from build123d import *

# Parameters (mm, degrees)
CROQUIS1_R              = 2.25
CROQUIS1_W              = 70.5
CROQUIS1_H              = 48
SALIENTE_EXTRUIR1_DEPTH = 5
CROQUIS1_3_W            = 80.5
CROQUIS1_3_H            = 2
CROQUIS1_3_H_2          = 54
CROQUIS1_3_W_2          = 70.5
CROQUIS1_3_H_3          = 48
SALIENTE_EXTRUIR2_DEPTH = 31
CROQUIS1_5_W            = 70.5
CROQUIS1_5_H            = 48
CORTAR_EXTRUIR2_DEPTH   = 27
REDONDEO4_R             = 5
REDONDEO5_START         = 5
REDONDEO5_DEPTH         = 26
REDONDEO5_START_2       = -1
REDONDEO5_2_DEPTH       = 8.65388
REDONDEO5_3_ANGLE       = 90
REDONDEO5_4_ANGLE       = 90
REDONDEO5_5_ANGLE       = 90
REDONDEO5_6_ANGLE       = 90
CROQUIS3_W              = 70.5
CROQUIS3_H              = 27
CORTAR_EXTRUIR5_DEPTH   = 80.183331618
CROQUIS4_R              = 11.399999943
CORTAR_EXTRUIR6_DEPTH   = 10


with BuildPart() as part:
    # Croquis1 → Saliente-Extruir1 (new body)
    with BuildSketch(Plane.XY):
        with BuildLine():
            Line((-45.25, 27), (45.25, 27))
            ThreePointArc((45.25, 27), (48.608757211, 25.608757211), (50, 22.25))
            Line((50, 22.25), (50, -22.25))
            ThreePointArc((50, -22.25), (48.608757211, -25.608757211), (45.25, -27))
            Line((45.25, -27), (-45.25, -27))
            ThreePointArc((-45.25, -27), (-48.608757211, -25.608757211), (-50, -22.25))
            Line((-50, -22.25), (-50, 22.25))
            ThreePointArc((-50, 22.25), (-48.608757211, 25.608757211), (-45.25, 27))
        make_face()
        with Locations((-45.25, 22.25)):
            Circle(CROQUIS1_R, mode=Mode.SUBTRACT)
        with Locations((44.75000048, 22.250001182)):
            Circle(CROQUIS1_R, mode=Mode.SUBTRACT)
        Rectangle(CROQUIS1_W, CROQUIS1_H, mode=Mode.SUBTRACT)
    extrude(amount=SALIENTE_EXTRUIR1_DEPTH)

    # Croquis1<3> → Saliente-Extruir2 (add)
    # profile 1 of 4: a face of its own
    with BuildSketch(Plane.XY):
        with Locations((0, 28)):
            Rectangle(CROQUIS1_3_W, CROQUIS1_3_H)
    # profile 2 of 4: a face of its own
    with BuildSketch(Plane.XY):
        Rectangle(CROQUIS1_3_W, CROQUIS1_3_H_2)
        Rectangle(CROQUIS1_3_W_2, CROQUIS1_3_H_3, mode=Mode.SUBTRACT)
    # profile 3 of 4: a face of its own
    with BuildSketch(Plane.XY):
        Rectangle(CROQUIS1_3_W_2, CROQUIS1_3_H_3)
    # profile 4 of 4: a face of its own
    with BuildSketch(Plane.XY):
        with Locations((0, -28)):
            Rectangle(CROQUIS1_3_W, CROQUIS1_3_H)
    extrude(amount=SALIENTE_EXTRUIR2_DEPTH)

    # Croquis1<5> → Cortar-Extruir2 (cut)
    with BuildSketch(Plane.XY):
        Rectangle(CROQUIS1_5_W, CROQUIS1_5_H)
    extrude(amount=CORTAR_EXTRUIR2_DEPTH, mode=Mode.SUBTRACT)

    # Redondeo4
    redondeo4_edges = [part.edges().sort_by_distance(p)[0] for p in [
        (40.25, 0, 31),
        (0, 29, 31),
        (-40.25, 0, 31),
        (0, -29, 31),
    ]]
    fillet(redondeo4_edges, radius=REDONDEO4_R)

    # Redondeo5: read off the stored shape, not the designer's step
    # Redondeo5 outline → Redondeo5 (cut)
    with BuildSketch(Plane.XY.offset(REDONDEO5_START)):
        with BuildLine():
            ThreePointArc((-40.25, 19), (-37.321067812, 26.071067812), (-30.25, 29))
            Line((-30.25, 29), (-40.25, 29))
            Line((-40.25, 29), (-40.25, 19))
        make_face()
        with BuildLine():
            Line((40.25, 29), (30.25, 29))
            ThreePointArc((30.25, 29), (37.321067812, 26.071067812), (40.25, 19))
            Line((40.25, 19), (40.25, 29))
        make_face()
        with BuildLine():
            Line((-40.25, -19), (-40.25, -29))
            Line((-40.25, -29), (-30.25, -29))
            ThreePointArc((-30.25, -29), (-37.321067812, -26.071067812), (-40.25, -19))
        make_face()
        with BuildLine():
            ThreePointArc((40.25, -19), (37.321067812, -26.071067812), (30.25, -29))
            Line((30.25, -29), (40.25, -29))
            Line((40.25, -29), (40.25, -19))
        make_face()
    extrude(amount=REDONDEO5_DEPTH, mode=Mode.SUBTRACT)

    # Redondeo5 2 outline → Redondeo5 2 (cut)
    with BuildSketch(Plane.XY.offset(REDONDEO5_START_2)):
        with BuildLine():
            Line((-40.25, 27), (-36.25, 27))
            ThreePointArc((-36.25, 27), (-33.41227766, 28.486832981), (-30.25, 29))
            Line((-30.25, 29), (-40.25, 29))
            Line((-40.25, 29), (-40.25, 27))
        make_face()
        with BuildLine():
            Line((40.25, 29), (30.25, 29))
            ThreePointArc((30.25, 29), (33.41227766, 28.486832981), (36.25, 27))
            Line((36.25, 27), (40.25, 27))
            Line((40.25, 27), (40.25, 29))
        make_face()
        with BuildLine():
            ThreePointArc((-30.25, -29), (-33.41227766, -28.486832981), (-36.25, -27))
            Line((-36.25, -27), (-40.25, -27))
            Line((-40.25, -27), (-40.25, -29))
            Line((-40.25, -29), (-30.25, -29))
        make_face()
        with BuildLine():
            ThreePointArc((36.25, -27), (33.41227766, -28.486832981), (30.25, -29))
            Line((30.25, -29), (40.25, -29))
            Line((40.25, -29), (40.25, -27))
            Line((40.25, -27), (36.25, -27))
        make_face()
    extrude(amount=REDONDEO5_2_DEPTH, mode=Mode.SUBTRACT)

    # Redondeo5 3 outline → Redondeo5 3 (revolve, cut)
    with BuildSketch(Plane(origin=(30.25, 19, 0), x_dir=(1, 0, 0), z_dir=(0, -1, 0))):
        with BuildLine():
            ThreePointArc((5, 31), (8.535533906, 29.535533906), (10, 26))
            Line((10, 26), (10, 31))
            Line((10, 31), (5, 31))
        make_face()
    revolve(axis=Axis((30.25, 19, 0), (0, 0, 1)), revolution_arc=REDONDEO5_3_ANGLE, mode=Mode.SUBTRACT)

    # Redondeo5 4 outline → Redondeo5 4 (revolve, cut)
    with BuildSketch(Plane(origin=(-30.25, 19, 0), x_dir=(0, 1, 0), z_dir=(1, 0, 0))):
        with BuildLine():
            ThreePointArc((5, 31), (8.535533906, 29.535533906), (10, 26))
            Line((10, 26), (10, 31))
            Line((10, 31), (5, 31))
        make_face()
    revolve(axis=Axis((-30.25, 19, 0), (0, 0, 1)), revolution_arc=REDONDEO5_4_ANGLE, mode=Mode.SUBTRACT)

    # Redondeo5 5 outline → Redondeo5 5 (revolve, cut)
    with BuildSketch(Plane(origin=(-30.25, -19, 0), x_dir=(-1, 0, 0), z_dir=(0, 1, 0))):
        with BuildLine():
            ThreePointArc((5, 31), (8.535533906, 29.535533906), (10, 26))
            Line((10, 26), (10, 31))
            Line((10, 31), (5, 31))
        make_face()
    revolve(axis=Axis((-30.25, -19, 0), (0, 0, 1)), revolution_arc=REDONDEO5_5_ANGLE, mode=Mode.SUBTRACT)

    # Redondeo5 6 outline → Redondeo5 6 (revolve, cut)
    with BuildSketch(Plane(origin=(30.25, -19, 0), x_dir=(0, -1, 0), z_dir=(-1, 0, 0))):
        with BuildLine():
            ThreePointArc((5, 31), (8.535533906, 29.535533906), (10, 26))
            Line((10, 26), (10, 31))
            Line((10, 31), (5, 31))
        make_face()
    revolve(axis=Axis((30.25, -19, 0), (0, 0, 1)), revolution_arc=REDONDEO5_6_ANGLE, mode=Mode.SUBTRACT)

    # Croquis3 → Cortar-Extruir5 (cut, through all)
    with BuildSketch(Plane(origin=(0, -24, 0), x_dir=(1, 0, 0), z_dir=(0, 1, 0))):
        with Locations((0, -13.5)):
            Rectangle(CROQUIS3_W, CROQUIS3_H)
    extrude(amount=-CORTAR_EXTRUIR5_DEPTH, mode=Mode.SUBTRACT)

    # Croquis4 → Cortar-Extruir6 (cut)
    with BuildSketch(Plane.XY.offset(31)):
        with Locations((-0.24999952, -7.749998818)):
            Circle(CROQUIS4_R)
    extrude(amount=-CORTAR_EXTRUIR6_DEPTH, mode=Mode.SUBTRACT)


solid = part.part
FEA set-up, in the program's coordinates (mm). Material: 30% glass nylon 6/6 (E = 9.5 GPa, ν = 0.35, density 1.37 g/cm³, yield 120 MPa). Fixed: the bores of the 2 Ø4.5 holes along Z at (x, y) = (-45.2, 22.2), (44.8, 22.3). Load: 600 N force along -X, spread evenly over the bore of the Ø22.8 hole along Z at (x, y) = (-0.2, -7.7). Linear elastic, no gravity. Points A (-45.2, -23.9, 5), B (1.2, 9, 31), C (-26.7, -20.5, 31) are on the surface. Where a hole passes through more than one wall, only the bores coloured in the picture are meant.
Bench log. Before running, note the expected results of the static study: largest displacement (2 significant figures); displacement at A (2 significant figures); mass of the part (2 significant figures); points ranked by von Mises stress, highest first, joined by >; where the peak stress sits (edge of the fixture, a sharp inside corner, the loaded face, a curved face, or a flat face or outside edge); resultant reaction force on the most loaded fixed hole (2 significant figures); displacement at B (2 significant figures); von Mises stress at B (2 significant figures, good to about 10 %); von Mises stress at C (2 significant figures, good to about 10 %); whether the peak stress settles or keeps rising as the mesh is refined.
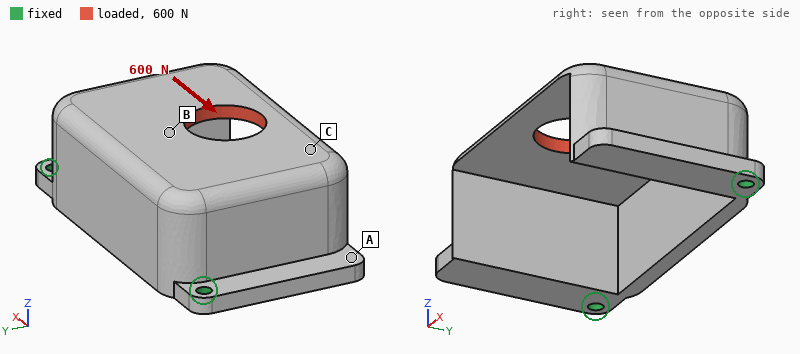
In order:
0.63 mm
0.38 mm
60 g
C > B > A
edge of the fixture
390 N
0.14 mm
7.2 MPa
12 MPa
keeps rising
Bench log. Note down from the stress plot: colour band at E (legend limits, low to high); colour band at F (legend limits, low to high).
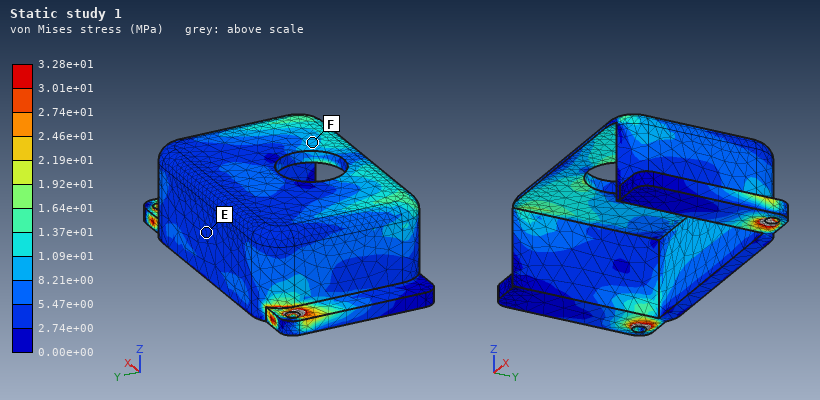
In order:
2.74e+00 to 5.47e+00 MPa
8.21e+00 to 1.09e+01 MPa
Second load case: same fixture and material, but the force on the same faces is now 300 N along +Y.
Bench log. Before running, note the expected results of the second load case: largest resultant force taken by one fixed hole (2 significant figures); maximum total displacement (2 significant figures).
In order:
150 N
0.73 mm
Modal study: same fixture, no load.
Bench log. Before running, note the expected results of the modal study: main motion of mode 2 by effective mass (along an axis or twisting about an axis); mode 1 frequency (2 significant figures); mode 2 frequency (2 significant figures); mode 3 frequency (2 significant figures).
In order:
along X
550 Hz
900 Hz
1900 Hz
